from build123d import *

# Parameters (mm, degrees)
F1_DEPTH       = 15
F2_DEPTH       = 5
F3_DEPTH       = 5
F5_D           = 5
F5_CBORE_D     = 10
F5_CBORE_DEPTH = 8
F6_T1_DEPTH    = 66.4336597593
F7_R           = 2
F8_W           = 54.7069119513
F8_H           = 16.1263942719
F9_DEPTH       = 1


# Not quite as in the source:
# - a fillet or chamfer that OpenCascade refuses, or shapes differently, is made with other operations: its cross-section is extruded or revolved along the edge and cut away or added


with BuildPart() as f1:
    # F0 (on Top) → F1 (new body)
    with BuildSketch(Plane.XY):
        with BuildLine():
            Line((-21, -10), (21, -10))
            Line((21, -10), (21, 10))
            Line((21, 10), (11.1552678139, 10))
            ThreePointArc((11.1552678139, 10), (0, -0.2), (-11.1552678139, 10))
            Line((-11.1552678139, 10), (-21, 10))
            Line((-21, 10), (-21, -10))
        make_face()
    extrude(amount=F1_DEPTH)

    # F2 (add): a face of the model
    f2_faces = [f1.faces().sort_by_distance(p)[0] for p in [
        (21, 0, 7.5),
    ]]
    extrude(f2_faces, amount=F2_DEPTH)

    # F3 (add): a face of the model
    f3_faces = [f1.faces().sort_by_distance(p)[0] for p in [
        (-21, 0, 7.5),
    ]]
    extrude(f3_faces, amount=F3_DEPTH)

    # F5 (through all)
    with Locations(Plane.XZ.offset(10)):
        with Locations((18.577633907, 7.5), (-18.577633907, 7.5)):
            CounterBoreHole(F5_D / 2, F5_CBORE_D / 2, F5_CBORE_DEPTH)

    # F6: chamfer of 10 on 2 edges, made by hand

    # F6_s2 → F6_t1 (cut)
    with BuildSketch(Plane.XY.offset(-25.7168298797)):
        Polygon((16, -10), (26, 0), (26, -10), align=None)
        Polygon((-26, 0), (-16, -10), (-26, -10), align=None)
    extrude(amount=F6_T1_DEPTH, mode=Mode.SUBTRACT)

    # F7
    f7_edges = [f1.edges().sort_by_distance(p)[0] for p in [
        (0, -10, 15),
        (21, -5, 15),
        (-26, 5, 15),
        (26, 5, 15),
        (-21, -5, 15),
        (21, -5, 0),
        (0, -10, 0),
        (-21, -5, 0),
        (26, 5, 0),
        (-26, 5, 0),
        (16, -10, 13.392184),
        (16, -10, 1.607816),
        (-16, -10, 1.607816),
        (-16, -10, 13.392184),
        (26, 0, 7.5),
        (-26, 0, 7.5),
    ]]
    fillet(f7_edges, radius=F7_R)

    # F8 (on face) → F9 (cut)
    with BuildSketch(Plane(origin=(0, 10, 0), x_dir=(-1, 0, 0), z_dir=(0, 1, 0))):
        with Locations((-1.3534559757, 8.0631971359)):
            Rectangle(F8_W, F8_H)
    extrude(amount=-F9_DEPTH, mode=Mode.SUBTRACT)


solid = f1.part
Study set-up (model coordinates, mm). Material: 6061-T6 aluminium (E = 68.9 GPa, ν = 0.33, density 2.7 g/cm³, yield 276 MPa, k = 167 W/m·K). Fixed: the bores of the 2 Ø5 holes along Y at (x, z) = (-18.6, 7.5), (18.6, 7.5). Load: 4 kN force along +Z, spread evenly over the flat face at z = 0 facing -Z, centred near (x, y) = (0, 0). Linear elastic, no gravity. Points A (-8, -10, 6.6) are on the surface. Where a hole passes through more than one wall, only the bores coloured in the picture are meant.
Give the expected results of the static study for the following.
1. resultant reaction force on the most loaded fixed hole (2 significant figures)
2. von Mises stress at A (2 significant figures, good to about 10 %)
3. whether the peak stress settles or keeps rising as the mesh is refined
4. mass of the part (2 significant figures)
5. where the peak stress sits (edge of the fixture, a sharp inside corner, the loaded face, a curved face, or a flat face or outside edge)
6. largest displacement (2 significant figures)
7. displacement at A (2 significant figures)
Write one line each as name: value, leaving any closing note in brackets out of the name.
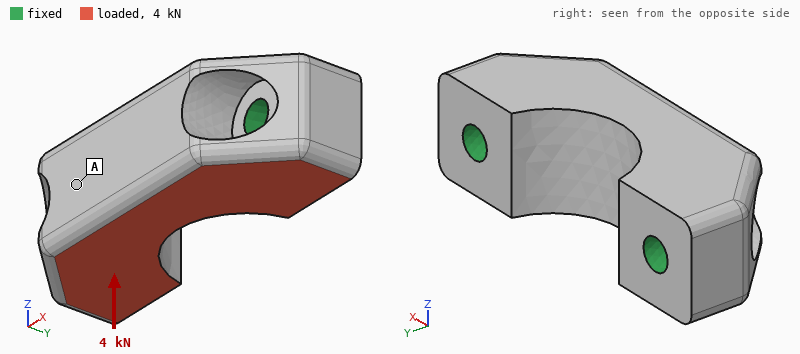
resultant reaction force on the most loaded fixed hole: 2.0 kN
von Mises stress at A: 11 MPa
whether the peak stress settles or keeps rising as the mesh is refined: keeps rising
mass of the part: 26 g
where the peak stress sits: edge of the fixture
largest displacement: 12 µm
displacement at A: 10 µm
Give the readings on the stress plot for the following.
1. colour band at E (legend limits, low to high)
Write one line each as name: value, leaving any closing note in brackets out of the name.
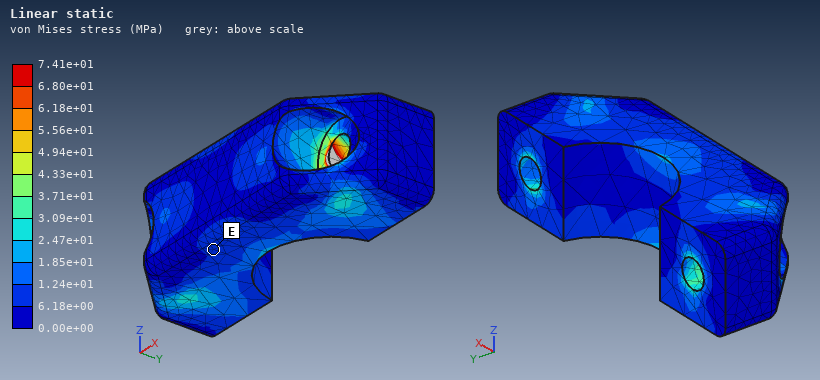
colour band at E: 6.18e+00 to 1.24e+01 MPa
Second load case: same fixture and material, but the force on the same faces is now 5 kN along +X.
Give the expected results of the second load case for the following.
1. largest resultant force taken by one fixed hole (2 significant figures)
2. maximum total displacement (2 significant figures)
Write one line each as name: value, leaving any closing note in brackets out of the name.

largest resultant force taken by one fixed hole: 2.6 kN
maximum total displacement: 6.7 µm
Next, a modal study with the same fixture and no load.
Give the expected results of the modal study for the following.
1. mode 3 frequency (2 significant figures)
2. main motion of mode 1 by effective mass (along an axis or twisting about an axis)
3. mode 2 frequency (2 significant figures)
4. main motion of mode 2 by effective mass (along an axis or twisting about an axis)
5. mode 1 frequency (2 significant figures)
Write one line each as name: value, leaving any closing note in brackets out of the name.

mode 3 frequency: 41 kHz
main motion of mode 1 by effective mass: along Z
mode 2 frequency: 33 kHz
main motion of mode 2 by effective mass: along Y
mode 1 frequency: 20 kHz
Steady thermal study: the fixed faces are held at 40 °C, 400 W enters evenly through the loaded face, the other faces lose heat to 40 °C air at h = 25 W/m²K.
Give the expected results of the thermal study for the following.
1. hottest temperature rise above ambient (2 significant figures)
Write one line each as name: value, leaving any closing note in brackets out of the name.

hottest temperature rise above ambient: 70 K
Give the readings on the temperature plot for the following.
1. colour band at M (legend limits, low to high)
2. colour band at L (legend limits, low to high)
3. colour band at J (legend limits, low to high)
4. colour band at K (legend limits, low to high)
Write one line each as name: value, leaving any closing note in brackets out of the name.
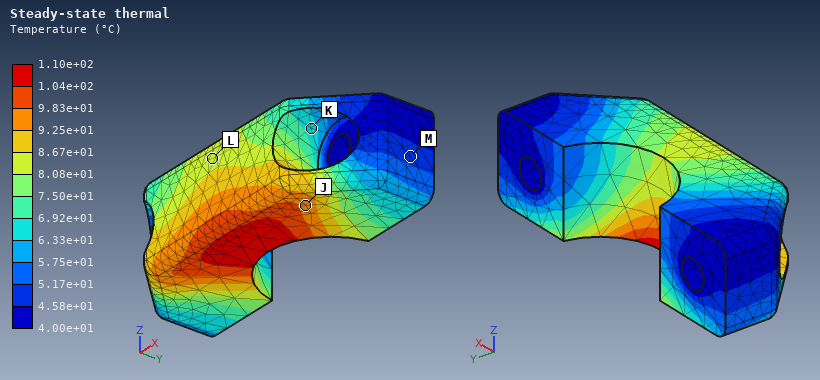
colour band at M: 4.58e+01 to 5.17e+01 °C
colour band at L: 8.08e+01 to 8.67e+01 °C
colour band at J: 9.25e+01 to 9.83e+01 °C
colour band at K: 6.33e+01 to 6.92e+01 °C
